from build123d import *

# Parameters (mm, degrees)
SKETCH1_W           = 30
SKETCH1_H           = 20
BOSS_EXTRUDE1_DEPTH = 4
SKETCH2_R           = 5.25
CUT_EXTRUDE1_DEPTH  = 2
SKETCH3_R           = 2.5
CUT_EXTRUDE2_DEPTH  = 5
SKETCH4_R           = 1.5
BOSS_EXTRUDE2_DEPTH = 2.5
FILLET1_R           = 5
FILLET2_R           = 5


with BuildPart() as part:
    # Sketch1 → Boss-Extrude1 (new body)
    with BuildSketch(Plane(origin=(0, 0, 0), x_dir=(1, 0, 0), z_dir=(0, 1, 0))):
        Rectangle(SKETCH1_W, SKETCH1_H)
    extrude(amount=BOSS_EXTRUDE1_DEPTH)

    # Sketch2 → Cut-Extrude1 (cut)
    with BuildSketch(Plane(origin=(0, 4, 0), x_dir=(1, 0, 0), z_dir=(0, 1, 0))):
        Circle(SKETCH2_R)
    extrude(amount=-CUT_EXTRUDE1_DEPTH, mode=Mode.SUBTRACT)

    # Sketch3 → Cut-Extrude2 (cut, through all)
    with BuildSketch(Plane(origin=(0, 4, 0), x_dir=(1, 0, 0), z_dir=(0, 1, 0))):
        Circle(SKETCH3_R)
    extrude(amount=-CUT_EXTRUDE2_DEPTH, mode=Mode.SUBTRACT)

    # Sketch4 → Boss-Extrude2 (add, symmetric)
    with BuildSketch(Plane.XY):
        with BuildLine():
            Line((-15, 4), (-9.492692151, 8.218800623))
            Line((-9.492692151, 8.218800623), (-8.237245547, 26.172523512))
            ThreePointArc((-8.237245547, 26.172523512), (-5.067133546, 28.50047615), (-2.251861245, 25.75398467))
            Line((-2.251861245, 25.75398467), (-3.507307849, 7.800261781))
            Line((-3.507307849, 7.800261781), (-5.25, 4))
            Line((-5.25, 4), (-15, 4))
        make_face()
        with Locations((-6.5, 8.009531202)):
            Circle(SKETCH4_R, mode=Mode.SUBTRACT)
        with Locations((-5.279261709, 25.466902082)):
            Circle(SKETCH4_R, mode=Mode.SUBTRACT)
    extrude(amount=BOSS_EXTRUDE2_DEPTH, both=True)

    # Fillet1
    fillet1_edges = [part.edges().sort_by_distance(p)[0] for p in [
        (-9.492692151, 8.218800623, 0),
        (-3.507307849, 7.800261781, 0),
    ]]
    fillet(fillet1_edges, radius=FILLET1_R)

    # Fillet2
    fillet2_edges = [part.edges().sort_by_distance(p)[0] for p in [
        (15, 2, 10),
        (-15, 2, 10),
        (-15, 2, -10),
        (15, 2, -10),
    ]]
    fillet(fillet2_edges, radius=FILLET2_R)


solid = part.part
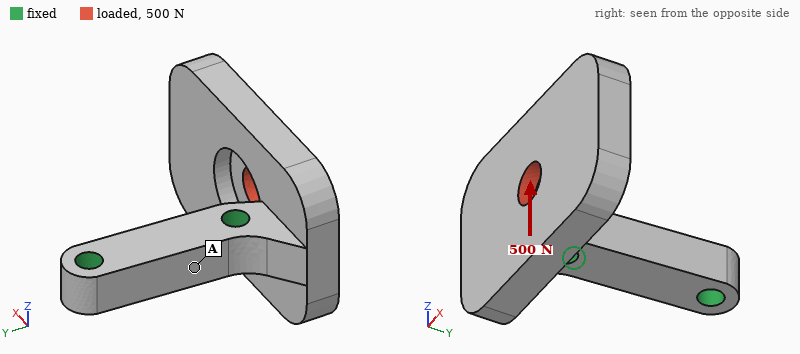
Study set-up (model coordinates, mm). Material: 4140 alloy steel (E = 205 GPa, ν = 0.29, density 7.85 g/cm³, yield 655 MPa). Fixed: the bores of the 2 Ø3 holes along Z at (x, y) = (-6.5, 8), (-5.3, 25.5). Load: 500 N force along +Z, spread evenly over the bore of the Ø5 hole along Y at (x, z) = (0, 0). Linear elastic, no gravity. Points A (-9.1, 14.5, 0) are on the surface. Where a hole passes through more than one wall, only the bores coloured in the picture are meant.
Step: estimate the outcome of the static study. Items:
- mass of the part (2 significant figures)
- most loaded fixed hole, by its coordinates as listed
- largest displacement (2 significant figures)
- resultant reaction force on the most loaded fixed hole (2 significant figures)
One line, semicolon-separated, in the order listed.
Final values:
22 g; (-6.5, 8); 40 µm; 500 N
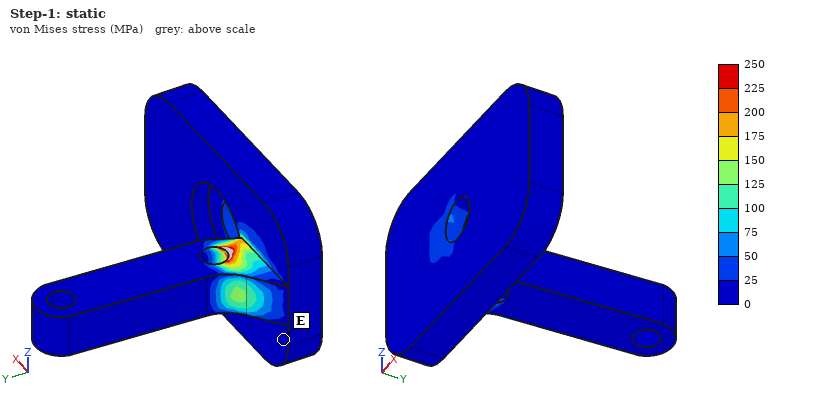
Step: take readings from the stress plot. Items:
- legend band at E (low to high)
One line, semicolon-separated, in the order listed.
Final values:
0 to 25 MPa
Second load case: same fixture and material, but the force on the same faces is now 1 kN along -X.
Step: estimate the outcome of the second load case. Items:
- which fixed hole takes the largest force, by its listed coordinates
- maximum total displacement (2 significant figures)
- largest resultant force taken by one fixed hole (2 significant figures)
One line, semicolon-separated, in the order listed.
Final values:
(-6.5, 8); 38 µm; 1.1 kN
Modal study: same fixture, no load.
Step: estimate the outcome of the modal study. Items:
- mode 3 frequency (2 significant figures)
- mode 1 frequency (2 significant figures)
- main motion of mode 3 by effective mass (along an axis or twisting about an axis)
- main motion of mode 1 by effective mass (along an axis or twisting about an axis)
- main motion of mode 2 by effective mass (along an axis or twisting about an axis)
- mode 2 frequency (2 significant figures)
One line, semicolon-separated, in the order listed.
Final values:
8400 Hz; 4000 Hz; twisting about X; along Y; along Z; 4800 Hz
